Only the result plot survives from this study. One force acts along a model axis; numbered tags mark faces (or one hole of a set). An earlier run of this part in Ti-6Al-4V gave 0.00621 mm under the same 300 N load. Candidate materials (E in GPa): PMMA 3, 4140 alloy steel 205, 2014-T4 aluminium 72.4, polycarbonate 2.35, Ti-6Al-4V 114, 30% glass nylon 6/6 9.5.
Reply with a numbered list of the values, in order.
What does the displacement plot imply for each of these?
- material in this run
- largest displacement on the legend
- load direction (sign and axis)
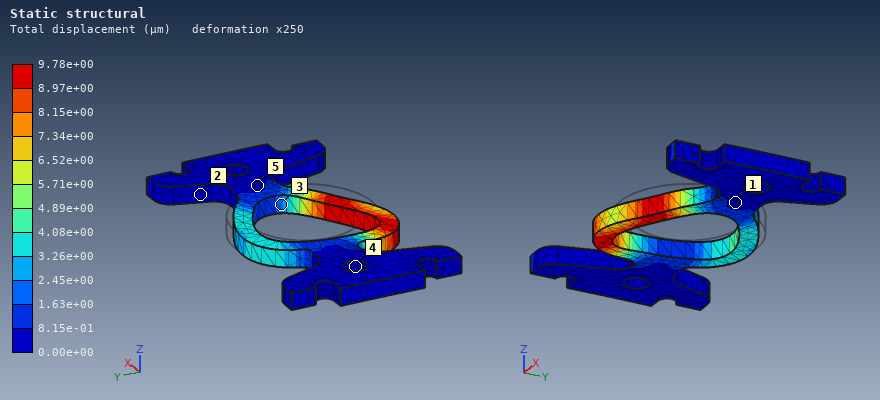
1. 2014-T4 aluminium
2. 9.78e+00 µm
3. -X
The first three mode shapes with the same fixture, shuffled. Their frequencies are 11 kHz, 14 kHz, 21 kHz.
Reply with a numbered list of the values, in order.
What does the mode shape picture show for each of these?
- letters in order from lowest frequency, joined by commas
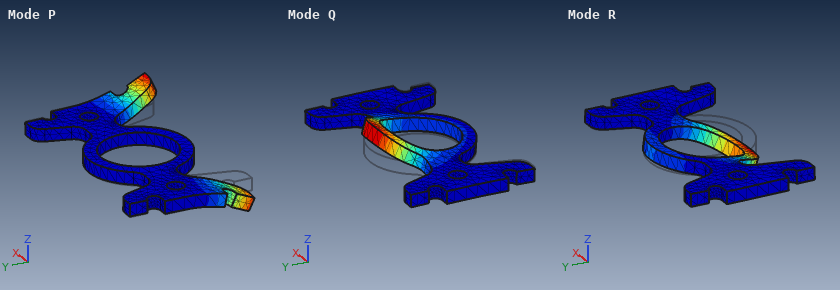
1. R, Q, P
